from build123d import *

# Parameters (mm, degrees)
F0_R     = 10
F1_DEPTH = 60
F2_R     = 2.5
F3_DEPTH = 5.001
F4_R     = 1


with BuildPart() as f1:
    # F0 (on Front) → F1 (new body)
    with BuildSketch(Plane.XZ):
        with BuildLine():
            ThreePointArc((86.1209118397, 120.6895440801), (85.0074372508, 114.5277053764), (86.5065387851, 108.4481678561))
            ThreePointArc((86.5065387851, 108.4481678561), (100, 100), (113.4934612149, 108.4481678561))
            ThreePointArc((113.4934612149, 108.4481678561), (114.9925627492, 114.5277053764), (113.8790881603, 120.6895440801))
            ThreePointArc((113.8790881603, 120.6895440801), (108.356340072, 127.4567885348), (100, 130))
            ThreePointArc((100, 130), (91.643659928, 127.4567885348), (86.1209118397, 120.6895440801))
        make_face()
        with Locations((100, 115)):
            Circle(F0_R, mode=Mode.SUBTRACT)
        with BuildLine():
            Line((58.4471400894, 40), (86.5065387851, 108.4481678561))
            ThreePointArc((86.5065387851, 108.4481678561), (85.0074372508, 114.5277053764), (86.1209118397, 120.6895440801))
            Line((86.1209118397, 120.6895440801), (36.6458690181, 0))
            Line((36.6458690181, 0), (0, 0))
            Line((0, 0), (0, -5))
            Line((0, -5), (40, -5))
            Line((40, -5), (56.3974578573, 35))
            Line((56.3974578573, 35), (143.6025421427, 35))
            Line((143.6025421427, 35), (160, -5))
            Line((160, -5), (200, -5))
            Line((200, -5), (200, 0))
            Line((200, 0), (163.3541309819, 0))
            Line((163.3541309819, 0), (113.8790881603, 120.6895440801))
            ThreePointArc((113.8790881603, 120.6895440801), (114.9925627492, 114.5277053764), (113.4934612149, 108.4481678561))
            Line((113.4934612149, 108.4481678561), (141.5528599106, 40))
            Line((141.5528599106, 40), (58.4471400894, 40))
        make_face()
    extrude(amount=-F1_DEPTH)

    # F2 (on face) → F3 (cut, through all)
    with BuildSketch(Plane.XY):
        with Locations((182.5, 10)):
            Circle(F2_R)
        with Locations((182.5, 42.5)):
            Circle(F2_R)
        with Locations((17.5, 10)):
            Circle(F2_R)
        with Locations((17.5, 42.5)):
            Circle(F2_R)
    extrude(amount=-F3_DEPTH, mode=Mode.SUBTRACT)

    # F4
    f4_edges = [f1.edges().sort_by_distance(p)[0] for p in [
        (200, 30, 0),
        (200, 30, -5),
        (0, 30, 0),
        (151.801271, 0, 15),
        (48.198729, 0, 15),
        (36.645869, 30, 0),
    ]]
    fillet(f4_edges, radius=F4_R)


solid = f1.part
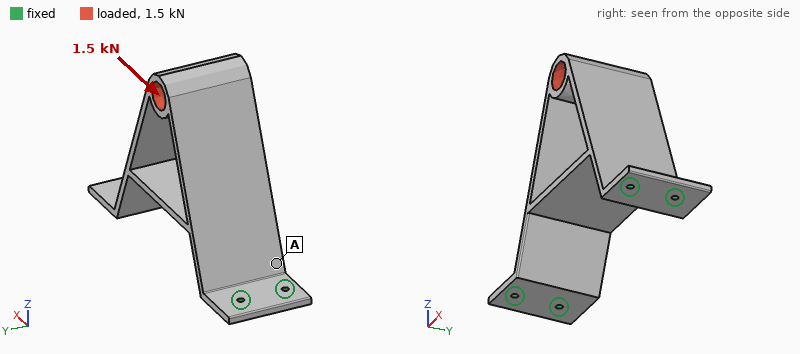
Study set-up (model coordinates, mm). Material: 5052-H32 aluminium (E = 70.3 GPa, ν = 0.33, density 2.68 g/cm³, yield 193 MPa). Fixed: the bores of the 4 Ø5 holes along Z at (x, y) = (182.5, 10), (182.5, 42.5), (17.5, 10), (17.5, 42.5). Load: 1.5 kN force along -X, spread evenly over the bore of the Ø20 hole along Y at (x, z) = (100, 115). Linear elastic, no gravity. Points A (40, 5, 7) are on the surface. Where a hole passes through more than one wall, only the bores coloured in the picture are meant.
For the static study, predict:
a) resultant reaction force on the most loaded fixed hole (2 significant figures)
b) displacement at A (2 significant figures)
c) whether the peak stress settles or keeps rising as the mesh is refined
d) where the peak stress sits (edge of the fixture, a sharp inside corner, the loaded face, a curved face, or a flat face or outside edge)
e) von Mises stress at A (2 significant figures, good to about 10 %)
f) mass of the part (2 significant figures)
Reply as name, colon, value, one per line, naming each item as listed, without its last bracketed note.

resultant reaction force on the most loaded fixed hole: 810 N
displacement at A: 0.053 mm
whether the peak stress settles or keeps rising as the mesh is refined: keeps rising
where the peak stress sits: edge of the fixture
von Mises stress at A: 36 MPa
mass of the part: 390 g
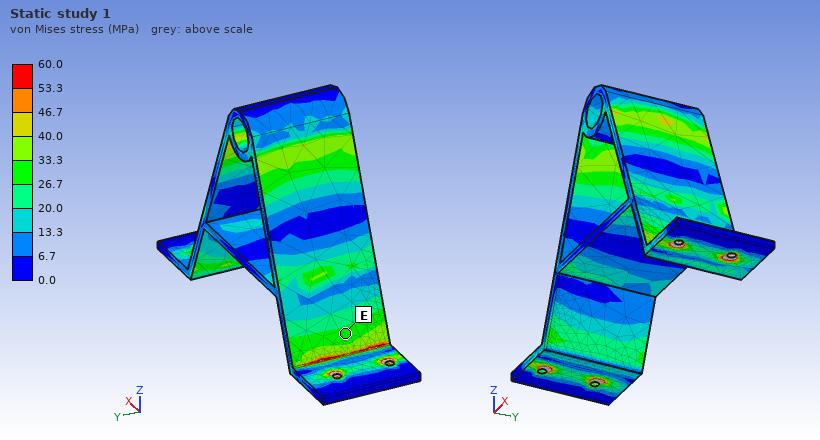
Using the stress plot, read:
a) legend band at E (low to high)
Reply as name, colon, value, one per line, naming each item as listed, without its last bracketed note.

legend band at E: 26.7 to 33.3 MPa
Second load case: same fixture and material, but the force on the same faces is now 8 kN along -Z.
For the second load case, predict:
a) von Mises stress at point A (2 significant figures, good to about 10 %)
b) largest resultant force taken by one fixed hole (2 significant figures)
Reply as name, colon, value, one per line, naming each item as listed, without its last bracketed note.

von Mises stress at point A: 92 MPa
largest resultant force taken by one fixed hole: 2.8 kN
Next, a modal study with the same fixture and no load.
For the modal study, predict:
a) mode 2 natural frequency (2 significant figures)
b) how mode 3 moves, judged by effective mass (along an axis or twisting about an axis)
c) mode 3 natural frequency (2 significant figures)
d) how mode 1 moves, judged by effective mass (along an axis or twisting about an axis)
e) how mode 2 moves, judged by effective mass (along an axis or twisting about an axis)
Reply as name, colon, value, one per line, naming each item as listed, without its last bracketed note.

mode 2 natural frequency: 840 Hz
how mode 3 moves, judged by effective mass: twisting about Y
mode 3 natural frequency: 1200 Hz
how mode 1 moves, judged by effective mass: along Y
how mode 2 moves, judged by effective mass: along X
